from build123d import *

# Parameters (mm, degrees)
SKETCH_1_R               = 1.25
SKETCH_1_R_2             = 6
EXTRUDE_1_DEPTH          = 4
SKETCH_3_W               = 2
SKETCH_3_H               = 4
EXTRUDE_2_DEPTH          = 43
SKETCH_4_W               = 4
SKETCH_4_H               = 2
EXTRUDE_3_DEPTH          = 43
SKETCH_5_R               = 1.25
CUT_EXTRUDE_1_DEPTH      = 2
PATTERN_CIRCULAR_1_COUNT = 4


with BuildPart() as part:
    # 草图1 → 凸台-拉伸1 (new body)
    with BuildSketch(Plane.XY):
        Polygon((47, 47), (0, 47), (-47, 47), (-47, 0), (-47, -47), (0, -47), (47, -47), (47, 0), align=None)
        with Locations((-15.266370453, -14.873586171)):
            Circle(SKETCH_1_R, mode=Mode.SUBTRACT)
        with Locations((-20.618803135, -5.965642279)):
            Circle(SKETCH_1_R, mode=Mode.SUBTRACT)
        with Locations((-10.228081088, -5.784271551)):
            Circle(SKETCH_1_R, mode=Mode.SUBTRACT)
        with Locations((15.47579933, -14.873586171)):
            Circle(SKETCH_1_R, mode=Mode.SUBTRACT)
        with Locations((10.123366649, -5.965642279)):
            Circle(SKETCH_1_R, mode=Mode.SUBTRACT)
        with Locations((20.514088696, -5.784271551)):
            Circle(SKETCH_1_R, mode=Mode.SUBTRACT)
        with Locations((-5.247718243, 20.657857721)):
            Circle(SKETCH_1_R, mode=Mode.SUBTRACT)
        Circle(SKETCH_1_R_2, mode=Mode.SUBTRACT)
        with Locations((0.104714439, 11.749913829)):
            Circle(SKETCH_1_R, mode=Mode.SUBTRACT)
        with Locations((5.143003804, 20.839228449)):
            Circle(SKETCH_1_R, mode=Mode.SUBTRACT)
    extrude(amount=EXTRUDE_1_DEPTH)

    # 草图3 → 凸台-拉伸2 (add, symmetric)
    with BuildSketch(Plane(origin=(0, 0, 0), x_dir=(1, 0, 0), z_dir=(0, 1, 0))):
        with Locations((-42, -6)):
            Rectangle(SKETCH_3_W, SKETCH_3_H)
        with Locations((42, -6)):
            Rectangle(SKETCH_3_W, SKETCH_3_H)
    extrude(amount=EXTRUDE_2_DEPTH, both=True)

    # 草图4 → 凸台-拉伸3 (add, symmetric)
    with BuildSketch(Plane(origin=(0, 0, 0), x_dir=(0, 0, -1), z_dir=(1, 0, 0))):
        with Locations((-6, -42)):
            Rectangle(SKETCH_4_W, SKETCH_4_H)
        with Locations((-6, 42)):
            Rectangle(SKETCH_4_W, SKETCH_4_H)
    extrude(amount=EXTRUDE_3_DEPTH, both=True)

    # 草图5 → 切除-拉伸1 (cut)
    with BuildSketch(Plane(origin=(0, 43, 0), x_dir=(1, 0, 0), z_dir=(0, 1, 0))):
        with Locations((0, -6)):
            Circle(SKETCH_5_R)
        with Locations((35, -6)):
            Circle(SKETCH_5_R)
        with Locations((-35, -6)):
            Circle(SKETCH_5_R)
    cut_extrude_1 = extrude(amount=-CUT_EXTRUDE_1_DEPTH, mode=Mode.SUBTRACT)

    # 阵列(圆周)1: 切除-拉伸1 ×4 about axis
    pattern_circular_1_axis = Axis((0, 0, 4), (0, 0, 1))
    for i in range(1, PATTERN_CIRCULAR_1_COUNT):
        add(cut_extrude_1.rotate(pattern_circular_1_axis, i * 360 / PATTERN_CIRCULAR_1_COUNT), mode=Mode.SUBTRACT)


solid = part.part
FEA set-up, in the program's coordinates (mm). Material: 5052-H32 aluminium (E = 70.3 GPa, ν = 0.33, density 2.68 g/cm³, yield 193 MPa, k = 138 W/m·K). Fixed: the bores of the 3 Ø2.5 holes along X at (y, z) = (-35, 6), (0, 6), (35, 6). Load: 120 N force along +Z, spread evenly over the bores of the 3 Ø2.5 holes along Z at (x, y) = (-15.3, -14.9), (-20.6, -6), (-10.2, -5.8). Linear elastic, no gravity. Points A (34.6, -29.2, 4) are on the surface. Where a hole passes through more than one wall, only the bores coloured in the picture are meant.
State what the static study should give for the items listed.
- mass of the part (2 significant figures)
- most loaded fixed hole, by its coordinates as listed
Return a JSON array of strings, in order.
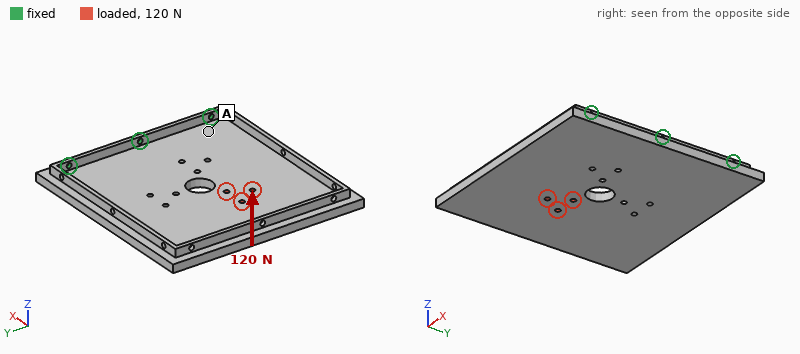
["100 g", "(0, 6)"]
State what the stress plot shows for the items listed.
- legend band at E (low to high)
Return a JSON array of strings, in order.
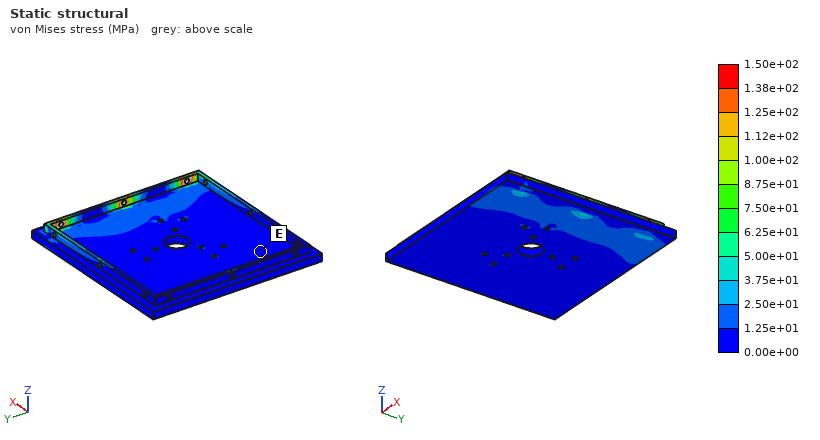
["0.00e+00 to 1.25e+01 MPa"]
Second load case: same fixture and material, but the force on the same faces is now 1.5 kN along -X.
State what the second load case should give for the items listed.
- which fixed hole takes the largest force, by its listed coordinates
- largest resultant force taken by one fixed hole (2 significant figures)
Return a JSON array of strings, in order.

["(-35, 6)", "690 N"]
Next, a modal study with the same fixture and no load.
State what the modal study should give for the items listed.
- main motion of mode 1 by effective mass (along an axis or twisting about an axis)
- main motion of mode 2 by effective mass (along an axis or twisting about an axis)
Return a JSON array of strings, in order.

["along Z", "twisting about X"]
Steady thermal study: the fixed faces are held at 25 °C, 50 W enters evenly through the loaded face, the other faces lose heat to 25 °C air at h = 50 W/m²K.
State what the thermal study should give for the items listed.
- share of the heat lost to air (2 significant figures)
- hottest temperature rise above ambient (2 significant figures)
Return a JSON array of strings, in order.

["56 %", "61 K"]
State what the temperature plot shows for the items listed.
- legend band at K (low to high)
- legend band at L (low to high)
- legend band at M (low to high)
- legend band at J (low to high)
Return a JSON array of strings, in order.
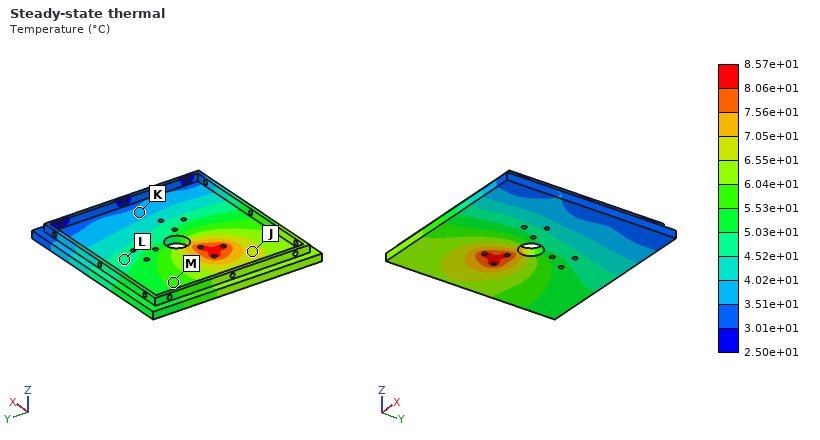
["3.51e+01 to 4.02e+01 °C", "4.52e+01 to 5.03e+01 °C", "5.53e+01 to 6.04e+01 °C", "6.55e+01 to 7.05e+01 °C"]
